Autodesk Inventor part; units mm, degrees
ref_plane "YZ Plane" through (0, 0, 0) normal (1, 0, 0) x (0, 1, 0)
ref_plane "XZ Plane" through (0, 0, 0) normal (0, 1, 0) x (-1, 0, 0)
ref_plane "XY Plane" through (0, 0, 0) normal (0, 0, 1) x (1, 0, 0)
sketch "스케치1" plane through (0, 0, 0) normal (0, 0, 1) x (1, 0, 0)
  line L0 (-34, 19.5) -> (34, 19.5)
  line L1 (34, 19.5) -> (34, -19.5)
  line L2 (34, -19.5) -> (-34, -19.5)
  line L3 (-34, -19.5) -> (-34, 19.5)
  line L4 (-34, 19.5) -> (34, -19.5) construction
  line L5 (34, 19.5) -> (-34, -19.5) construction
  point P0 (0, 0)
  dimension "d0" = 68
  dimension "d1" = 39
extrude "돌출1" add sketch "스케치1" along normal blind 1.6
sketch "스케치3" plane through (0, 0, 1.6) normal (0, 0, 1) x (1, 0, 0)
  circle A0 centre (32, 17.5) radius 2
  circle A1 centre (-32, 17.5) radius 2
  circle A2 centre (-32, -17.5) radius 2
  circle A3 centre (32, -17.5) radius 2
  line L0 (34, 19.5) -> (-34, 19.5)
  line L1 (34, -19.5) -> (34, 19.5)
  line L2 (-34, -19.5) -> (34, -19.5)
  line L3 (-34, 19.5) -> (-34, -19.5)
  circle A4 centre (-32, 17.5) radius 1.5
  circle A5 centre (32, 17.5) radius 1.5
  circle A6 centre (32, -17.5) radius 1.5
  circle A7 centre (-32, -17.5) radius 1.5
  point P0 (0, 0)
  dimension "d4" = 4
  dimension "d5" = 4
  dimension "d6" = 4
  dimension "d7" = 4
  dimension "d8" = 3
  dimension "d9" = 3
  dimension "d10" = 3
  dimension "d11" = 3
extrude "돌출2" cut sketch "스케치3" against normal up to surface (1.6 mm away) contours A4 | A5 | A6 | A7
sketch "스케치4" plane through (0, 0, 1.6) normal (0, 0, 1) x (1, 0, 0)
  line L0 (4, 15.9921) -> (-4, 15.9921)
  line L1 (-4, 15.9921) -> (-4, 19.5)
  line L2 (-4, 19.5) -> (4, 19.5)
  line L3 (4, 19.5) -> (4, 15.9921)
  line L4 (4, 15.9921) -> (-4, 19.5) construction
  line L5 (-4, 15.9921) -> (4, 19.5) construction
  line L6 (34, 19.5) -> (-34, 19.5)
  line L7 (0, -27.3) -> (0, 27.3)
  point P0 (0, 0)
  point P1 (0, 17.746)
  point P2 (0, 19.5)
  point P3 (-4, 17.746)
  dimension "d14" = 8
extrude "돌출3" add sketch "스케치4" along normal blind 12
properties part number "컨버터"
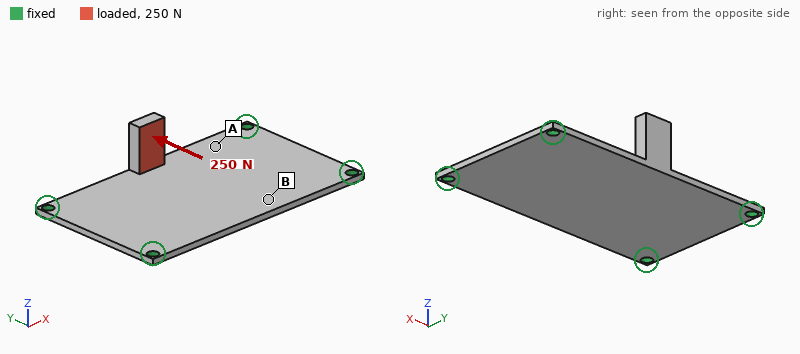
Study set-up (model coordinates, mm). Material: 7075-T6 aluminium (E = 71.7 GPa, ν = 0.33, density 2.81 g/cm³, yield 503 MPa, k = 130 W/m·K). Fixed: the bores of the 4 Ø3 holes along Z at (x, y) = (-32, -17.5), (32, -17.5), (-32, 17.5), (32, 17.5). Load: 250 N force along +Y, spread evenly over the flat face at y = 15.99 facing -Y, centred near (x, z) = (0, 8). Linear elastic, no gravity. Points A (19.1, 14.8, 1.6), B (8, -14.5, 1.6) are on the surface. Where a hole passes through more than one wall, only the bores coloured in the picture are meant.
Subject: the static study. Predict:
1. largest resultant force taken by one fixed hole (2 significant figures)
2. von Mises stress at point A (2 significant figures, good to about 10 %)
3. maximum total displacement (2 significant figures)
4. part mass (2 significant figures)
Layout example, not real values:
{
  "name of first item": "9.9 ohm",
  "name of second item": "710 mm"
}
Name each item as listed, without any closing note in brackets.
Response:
{
  "largest resultant force taken by one fixed hole": "94 N",
  "von Mises stress at point A": "69 MPa",
  "maximum total displacement": "0.52 mm",
  "part mass": "13 g"
}
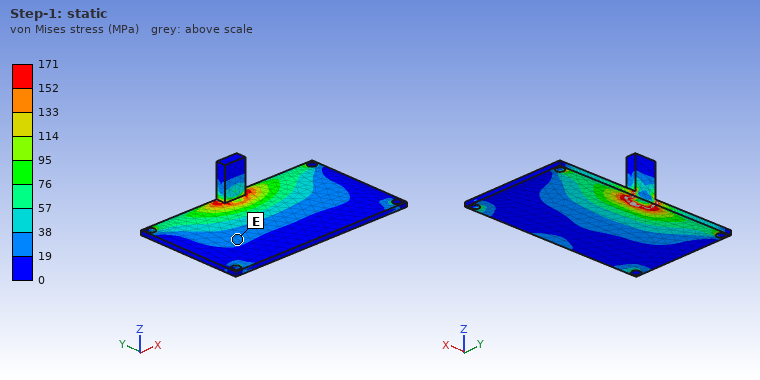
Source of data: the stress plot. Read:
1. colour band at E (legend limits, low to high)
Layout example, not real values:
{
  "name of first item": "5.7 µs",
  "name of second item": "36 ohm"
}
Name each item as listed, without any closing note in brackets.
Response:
{
  "colour band at E": "19 to 38 MPa"
}
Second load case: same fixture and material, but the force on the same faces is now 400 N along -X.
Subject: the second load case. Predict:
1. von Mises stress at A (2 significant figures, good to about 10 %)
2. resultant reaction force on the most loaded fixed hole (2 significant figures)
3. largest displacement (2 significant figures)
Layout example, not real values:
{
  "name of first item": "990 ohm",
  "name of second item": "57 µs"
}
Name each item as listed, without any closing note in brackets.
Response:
{
  "von Mises stress at A": "52 MPa",
  "resultant reaction force on the most loaded fixed hole": "140 N",
  "largest displacement": "0.35 mm"
}
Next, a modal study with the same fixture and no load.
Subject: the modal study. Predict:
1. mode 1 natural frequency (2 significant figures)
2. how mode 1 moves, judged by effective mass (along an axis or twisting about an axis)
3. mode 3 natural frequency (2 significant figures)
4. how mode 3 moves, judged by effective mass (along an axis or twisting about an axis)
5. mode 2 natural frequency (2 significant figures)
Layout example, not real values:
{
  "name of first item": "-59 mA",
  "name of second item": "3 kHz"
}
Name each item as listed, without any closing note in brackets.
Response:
{
  "mode 1 natural frequency": "1600 Hz",
  "how mode 1 moves, judged by effective mass": "along Z",
  "mode 3 natural frequency": "4400 Hz",
  "how mode 3 moves, judged by effective mass": "twisting about Y",
  "mode 2 natural frequency": "2500 Hz"
}
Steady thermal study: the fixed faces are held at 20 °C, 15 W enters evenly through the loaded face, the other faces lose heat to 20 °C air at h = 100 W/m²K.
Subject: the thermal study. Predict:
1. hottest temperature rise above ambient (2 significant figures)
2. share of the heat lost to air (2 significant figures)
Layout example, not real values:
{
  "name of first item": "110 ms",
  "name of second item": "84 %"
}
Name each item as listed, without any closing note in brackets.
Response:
{
  "hottest temperature rise above ambient": "72 K",
  "share of the heat lost to air": "51 %"
}
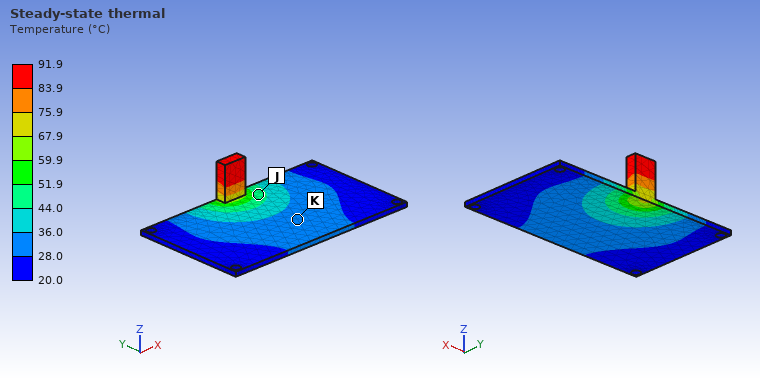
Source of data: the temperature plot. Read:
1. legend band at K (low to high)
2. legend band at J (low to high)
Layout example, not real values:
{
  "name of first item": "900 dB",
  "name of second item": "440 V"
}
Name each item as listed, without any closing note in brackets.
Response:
{
  "legend band at K": "28.0 to 36.0 °C",
  "legend band at J": "44.0 to 51.9 °C"
}
